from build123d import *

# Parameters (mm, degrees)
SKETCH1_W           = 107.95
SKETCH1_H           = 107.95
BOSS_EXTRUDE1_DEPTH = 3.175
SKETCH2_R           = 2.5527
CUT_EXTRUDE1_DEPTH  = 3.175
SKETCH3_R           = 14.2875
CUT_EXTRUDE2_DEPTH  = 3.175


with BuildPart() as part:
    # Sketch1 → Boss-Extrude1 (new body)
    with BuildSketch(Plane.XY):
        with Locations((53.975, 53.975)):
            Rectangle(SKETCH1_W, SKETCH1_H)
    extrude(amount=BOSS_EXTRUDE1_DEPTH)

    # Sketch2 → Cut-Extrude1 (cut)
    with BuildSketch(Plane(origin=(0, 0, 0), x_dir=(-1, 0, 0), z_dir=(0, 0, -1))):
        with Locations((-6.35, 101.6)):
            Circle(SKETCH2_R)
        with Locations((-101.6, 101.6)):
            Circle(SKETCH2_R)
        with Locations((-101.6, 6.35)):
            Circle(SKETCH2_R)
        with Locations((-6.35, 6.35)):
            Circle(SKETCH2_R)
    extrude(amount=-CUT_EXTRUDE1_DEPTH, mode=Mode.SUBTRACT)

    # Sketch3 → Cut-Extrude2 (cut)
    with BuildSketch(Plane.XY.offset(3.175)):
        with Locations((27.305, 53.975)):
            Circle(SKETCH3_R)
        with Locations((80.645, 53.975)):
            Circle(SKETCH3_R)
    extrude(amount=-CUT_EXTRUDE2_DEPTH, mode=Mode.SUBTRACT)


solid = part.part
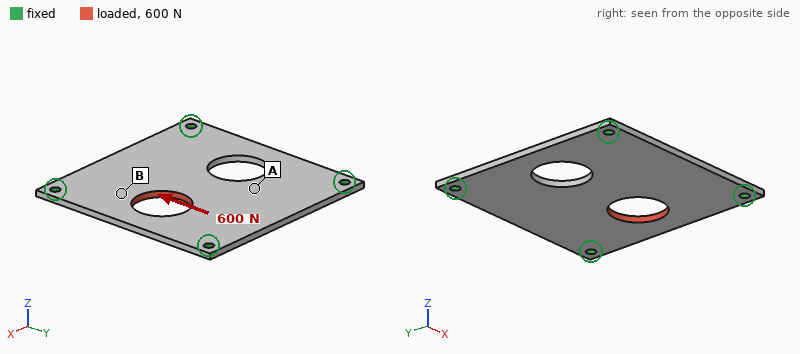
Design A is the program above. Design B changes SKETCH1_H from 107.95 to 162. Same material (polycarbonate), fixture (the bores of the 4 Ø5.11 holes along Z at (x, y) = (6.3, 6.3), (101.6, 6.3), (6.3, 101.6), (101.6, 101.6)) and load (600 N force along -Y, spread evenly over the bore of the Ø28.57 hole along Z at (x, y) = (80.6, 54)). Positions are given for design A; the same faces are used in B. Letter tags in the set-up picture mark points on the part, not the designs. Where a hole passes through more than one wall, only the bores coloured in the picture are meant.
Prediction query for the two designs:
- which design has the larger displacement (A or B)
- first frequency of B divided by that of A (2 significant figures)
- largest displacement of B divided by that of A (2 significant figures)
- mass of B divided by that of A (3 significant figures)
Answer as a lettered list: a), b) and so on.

a) A
b) 1.0
c) 0.74
d) 1.57
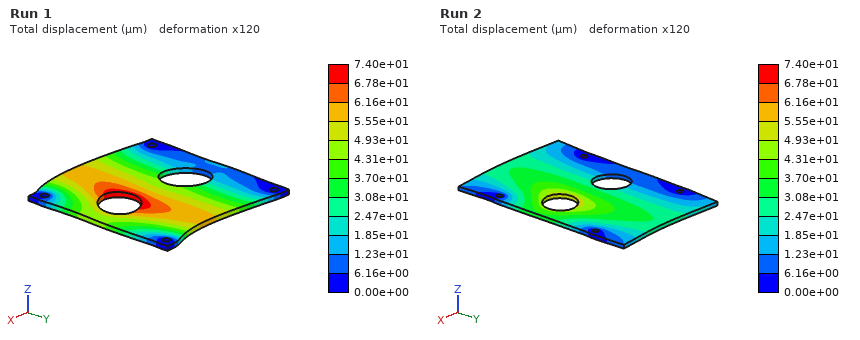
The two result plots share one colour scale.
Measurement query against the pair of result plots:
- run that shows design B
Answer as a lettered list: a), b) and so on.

a) Run 2
